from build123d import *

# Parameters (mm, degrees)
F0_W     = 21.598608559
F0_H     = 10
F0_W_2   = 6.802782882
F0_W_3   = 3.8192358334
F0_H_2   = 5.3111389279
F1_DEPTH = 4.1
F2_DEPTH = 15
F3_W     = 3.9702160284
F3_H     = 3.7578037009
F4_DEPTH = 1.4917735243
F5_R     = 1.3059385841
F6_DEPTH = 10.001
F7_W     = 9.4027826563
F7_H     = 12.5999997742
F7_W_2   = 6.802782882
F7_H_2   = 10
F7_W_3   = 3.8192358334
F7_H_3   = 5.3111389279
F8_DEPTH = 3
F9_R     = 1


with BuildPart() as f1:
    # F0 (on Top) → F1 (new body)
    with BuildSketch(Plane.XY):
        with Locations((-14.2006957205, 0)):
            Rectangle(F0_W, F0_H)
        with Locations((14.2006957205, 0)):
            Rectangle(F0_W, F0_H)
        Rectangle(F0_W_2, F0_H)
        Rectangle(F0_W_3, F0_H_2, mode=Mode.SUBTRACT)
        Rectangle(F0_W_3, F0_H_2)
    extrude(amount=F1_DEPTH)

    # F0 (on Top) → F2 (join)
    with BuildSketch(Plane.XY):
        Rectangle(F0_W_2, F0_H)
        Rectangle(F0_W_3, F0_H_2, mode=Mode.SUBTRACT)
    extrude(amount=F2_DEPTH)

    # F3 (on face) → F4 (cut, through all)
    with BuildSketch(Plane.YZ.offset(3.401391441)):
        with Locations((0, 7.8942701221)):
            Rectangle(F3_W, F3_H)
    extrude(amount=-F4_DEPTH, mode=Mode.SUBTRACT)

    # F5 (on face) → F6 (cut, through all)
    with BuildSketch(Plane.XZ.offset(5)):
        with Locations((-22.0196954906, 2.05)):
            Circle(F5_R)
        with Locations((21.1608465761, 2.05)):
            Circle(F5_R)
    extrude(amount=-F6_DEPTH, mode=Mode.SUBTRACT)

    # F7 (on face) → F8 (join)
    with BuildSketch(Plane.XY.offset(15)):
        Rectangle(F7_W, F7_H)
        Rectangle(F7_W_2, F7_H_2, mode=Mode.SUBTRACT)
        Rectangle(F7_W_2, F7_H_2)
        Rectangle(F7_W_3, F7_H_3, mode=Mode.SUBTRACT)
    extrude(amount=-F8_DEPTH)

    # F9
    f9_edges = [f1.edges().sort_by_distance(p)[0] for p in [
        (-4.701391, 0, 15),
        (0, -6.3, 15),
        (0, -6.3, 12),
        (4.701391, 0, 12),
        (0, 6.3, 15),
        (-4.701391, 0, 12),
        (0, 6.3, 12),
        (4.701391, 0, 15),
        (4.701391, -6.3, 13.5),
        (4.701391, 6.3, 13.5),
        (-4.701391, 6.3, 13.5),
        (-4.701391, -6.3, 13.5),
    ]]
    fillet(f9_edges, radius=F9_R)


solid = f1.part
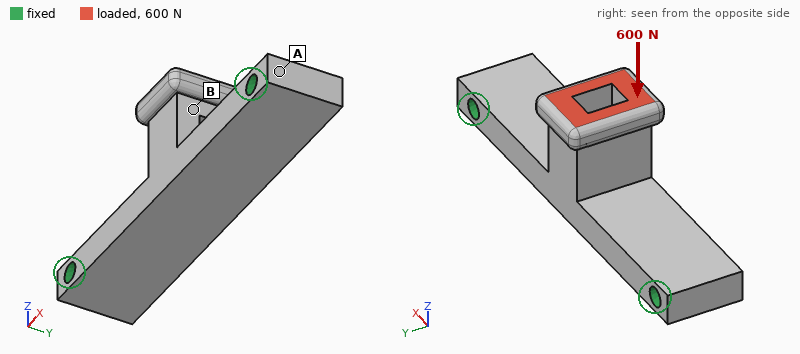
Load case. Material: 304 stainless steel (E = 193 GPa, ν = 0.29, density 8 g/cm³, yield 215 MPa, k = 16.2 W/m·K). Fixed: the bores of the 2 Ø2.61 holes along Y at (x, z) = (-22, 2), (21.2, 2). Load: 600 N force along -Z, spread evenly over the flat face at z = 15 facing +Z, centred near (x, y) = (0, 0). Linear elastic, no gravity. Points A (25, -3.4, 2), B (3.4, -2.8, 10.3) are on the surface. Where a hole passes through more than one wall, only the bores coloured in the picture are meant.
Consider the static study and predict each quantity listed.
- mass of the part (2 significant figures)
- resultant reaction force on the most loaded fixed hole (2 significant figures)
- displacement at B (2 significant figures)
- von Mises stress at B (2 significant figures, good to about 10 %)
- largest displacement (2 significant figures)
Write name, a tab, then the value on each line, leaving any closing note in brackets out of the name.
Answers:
mass of the part	21 g
resultant reaction force on the most loaded fixed hole	320 N
displacement at B	20 µm
von Mises stress at B	21 MPa
largest displacement	20 µm
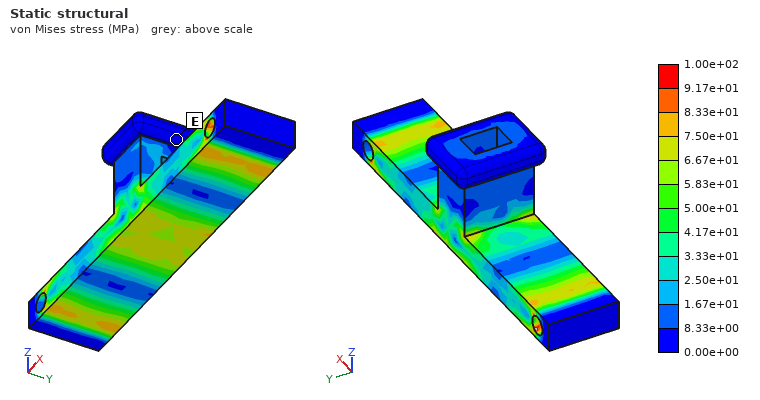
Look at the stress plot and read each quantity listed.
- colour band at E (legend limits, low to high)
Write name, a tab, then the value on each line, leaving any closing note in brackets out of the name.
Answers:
colour band at E	0.00e+00 to 8.33e+00 MPa
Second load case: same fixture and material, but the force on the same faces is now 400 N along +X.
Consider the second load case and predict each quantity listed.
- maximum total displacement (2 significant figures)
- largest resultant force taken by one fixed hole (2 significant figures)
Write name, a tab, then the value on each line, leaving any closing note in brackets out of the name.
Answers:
maximum total displacement	21 µm
largest resultant force taken by one fixed hole	270 N
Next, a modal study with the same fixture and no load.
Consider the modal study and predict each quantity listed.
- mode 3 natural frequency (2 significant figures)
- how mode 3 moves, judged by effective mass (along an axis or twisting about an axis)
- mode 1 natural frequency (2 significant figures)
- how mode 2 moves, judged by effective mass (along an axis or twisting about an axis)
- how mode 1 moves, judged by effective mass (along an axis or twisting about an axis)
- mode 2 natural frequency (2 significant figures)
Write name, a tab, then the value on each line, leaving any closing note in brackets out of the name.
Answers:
mode 3 natural frequency	14 kHz
how mode 3 moves, judged by effective mass	along X
mode 1 natural frequency	8000 Hz
how mode 2 moves, judged by effective mass	along Z
how mode 1 moves, judged by effective mass	along Y
mode 2 natural frequency	8500 Hz
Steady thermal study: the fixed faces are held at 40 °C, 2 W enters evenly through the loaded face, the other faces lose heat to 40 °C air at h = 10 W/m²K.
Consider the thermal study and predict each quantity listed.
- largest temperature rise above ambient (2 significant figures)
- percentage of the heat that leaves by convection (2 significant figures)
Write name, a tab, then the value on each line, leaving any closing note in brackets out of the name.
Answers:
largest temperature rise above ambient	52 K
percentage of the heat that leaves by convection	19 %
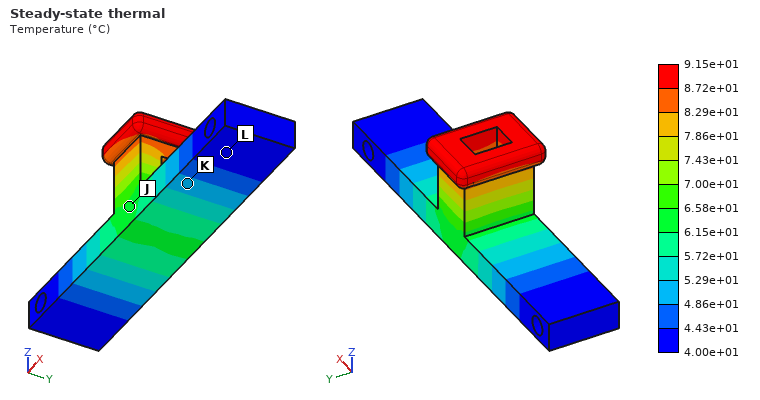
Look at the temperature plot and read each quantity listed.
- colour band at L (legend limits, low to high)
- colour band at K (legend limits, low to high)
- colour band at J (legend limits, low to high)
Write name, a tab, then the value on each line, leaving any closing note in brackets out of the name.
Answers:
colour band at L	4.00e+01 to 4.43e+01 °C
colour band at K	4.86e+01 to 5.29e+01 °C
colour band at J	6.15e+01 to 6.58e+01 °C
